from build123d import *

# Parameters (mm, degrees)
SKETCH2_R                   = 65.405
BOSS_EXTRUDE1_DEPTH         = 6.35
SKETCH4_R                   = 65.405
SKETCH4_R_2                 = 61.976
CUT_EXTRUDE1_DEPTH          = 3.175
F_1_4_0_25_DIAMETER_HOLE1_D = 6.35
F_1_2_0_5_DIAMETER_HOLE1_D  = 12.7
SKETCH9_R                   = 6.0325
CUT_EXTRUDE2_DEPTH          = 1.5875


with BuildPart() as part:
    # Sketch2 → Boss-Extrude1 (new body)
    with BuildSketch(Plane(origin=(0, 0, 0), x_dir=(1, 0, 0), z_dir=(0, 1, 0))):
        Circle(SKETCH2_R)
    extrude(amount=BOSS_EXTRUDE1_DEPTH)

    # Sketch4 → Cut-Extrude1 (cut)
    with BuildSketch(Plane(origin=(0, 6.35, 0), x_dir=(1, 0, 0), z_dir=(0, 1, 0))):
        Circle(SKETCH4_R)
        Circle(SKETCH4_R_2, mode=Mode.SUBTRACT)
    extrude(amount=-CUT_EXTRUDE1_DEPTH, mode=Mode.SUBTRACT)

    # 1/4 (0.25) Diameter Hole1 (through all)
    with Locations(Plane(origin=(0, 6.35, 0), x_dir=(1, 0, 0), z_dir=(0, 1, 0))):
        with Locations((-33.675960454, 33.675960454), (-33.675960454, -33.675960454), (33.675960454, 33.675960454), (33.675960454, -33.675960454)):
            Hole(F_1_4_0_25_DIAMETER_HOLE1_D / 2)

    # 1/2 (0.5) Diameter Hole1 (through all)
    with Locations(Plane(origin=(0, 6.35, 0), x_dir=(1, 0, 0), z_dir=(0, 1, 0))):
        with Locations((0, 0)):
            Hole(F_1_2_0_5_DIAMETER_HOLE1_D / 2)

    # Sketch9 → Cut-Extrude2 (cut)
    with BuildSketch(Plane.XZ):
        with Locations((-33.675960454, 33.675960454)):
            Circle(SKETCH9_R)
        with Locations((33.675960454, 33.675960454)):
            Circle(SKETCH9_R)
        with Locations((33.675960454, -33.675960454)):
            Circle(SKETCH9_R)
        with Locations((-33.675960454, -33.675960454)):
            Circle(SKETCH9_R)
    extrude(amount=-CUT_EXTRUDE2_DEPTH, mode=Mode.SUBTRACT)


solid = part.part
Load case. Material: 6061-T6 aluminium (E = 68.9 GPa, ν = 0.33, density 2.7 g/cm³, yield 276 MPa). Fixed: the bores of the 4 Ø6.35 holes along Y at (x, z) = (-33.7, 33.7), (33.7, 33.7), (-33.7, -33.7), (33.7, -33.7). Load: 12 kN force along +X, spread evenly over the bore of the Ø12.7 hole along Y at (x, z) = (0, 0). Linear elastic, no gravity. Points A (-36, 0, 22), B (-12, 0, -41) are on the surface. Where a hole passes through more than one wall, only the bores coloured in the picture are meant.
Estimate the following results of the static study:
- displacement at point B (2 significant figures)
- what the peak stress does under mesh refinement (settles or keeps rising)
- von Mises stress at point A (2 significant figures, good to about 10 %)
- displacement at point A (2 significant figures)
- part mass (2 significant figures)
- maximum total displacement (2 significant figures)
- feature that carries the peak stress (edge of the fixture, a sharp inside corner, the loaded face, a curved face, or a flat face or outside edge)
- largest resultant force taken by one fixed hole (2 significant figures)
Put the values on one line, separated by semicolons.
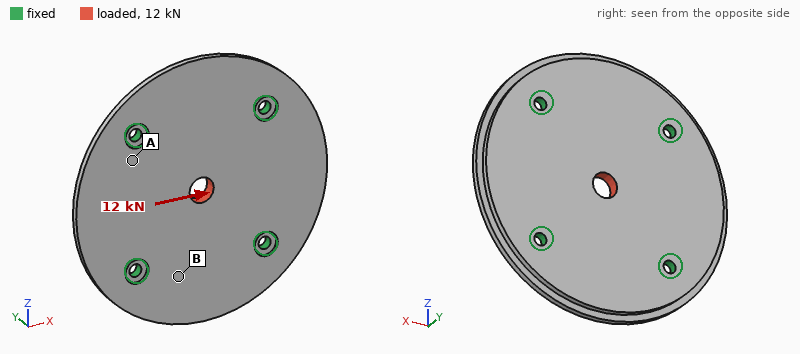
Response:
3.1 µm; keeps rising; 14 MPa; 6.4 µm; 210 g; 20 µm; edge of the fixture; 3.1 kN
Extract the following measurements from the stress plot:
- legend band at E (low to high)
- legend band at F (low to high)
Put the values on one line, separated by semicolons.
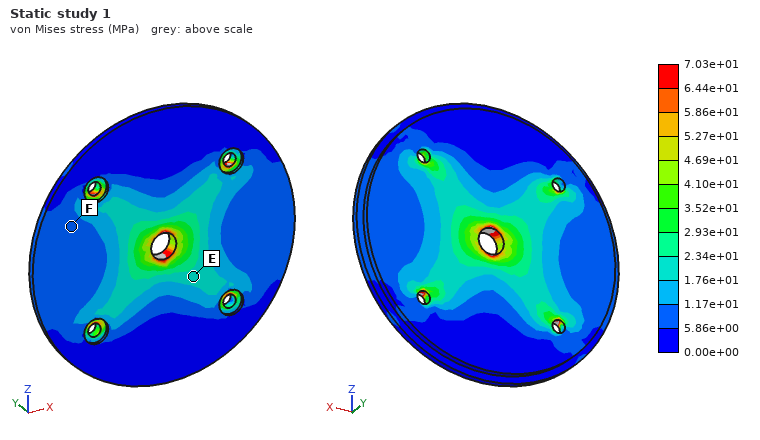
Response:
1.76e+01 to 2.34e+01 MPa; 5.86e+00 to 1.17e+01 MPa
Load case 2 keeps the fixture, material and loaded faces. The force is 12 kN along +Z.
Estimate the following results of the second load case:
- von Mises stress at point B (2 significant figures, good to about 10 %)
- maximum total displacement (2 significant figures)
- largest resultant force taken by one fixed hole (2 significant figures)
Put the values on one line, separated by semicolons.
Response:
8.6 MPa; 20 µm; 3.1 kN
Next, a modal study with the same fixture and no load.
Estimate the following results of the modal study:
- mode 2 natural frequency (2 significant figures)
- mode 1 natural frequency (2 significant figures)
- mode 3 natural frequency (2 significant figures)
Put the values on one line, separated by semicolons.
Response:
4200 Hz; 3800 Hz; 4200 Hz
